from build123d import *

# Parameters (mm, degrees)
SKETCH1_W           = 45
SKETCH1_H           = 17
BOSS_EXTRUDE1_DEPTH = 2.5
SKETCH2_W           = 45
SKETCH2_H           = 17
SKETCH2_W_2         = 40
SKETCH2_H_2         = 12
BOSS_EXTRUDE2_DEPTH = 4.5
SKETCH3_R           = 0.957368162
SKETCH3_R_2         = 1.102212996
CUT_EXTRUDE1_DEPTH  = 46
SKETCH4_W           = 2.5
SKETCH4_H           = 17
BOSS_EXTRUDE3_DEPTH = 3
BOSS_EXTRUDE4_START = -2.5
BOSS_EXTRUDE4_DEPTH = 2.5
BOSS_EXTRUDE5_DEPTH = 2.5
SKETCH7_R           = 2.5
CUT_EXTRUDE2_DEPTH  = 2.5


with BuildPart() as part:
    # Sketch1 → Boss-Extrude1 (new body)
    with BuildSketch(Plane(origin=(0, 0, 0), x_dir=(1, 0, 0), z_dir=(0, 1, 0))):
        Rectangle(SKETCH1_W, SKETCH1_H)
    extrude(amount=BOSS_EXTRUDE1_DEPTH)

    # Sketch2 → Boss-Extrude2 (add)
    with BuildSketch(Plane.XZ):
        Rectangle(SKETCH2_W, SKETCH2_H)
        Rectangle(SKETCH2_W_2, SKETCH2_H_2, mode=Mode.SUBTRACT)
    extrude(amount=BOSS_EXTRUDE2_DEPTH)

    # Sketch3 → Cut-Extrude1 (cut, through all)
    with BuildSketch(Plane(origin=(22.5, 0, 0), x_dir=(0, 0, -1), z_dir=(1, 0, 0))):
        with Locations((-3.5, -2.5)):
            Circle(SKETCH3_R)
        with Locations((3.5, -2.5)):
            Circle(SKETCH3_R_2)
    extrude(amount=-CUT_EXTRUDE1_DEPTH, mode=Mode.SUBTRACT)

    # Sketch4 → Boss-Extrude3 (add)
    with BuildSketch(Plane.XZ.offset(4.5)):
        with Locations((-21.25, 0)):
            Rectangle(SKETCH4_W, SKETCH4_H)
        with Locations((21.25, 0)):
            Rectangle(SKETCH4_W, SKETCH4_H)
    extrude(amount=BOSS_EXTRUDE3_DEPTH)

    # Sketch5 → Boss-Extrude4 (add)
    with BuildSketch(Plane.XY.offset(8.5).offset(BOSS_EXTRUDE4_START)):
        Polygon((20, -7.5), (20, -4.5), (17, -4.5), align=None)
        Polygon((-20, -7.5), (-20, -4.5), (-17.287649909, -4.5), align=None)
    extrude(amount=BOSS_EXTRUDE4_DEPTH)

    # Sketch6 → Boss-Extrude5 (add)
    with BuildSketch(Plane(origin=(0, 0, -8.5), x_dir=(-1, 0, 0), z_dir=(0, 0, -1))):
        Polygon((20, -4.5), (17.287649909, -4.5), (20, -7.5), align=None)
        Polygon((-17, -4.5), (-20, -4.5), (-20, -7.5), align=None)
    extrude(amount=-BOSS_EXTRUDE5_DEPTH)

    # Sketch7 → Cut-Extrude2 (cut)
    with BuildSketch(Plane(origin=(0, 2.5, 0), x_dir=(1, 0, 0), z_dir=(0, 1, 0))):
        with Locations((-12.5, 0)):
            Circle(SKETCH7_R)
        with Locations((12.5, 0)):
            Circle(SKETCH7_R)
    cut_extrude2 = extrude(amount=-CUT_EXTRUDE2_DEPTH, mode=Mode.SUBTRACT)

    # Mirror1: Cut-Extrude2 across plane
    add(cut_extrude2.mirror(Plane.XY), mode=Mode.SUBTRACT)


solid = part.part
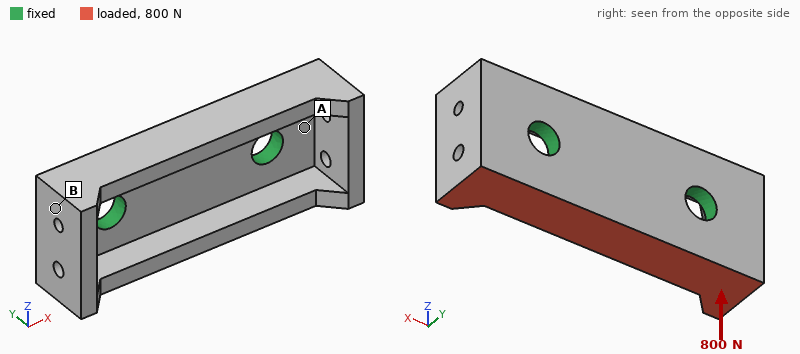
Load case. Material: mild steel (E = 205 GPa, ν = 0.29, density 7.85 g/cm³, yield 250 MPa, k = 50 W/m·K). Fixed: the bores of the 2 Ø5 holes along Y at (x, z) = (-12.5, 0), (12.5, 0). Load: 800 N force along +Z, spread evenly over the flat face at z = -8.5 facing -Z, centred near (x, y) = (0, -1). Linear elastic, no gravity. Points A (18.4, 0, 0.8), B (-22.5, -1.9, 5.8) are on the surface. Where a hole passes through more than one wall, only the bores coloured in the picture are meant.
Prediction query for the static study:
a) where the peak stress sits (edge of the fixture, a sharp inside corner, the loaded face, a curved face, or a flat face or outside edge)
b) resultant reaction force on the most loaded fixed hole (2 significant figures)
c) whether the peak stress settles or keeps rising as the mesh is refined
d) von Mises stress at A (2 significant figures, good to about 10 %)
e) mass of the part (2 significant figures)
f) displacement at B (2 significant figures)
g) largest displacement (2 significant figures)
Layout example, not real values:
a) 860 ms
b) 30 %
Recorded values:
a) edge of the fixture
b) 400 N
c) keeps rising
d) 18 MPa
e) 26 g
f) 2.5 µm
g) 6.5 µm
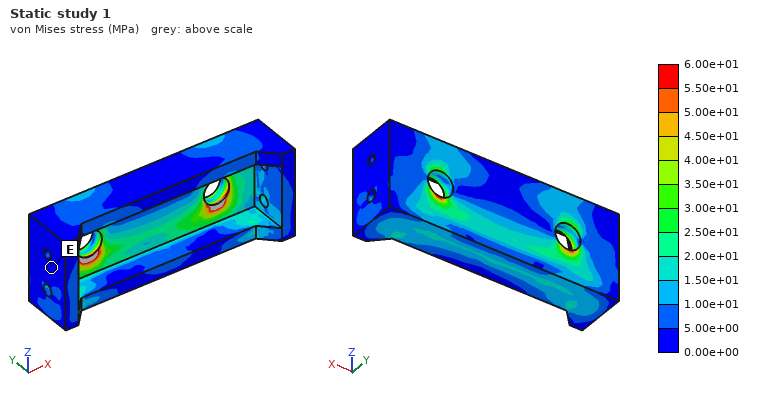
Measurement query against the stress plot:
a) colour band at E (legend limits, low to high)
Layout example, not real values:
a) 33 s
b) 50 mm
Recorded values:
a) 0.00e+00 to 5.00e+00 MPa
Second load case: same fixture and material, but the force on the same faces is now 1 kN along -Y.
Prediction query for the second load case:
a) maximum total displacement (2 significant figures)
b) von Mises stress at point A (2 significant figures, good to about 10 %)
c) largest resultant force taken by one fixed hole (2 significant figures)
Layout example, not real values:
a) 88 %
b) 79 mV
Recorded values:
a) 17 µm
b) 38 MPa
c) 500 N
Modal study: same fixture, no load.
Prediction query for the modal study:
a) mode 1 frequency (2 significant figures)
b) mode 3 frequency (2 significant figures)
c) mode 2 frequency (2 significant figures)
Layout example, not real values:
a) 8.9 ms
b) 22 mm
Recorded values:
a) 14 kHz
b) 18 kHz
c) 14 kHz
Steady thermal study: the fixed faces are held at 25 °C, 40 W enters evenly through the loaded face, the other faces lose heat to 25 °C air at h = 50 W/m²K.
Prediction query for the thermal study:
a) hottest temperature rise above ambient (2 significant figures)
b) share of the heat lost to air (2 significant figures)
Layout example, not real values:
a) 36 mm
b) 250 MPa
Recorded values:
a) 66 K
b) 8.8 %
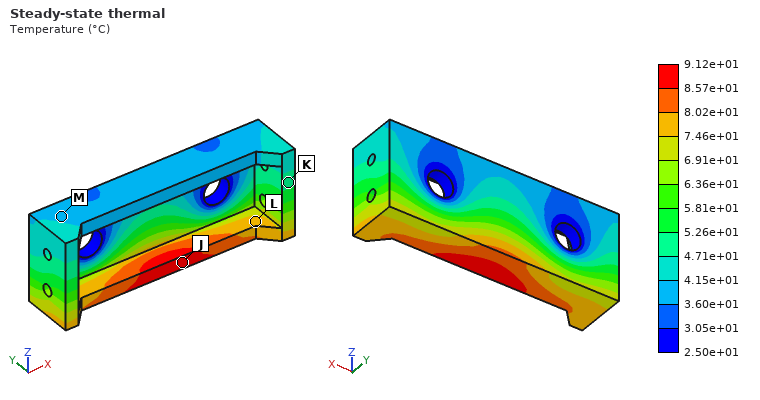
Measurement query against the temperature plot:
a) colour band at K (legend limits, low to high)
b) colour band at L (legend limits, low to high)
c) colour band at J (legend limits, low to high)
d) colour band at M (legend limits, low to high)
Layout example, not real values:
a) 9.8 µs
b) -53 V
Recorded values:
a) 4.71e+01 to 5.26e+01 °C
b) 7.46e+01 to 8.02e+01 °C
c) 8.57e+01 to 9.12e+01 °C
d) 3.60e+01 to 4.15e+01 °C
